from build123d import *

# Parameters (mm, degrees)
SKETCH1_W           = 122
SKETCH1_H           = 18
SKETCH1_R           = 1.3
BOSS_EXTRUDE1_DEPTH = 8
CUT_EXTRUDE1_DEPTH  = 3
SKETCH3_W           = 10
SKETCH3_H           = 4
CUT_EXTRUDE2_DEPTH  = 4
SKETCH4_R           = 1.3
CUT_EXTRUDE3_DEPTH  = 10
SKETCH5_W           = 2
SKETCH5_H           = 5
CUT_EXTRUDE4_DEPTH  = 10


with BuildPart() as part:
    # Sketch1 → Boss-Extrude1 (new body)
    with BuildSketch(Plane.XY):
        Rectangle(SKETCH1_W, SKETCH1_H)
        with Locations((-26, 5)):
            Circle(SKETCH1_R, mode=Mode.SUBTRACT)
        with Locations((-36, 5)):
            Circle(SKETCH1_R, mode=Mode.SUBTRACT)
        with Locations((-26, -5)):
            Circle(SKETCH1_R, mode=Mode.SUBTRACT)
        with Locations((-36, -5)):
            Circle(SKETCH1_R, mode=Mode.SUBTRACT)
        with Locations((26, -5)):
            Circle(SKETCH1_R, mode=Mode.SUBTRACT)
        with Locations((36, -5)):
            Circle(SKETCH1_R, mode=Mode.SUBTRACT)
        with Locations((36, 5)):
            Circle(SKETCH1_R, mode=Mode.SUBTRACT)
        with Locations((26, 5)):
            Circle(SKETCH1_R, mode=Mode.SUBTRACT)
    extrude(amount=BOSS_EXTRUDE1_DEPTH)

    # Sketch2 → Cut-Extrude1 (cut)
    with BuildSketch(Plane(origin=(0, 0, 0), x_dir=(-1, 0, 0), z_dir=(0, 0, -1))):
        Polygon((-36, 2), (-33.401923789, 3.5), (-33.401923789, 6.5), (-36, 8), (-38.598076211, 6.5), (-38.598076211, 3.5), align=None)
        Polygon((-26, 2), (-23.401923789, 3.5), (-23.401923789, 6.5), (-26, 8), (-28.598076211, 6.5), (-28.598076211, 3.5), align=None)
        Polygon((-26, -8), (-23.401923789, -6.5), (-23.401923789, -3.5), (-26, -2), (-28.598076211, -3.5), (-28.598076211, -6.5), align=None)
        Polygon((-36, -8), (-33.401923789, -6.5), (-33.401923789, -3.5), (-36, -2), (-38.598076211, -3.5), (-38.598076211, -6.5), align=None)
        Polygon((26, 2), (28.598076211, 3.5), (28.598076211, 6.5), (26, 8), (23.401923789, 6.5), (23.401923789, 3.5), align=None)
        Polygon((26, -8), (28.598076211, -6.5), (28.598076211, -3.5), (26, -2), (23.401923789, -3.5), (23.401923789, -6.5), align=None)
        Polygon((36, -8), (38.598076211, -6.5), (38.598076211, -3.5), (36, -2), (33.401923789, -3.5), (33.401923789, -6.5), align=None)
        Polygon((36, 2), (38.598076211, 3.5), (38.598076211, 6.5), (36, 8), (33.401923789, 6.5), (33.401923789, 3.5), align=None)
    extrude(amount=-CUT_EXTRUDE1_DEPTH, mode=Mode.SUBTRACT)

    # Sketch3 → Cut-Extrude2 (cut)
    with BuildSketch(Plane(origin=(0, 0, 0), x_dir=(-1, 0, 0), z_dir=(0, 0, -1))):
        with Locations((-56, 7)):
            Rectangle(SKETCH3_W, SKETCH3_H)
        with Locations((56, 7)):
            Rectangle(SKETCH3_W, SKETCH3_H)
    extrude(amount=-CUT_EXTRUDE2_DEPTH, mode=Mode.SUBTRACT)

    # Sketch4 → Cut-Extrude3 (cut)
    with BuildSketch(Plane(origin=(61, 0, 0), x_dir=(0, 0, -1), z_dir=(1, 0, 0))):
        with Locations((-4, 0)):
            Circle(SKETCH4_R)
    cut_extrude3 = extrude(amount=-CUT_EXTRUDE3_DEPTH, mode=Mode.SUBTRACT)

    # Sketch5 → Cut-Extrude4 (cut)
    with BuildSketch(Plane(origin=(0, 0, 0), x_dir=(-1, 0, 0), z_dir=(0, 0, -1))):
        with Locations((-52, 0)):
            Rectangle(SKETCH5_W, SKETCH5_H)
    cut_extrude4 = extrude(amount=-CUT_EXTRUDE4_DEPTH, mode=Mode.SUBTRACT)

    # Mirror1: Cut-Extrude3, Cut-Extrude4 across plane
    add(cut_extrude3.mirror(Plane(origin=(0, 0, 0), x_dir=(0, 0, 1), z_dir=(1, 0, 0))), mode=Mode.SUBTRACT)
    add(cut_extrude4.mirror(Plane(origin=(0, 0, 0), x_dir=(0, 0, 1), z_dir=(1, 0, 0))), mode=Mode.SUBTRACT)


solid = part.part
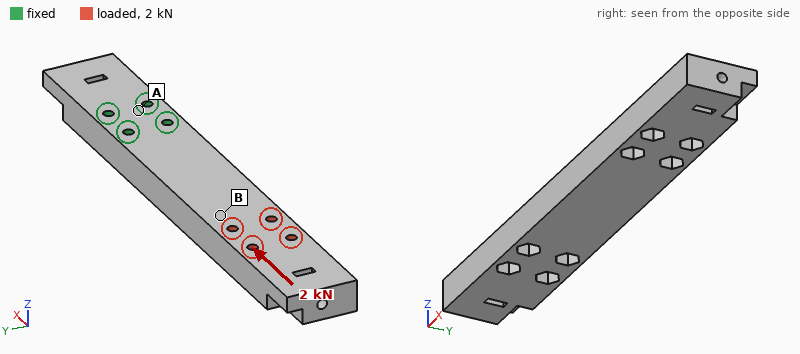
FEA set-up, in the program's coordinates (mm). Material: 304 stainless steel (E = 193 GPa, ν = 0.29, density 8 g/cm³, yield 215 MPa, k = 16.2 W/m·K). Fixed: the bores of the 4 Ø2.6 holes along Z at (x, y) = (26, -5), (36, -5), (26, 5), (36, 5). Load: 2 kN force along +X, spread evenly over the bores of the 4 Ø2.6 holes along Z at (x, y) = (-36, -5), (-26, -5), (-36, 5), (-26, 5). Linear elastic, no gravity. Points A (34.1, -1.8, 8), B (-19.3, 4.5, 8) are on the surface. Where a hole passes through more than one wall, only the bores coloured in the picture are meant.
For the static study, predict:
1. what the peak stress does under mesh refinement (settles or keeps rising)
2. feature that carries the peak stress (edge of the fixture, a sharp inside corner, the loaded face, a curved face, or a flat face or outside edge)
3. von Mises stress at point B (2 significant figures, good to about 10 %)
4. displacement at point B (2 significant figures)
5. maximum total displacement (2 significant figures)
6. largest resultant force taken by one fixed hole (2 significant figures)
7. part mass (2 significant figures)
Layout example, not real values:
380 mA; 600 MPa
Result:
keeps rising; edge of the fixture; 29 MPa; 21 µm; 65 µm; 880 N; 130 g
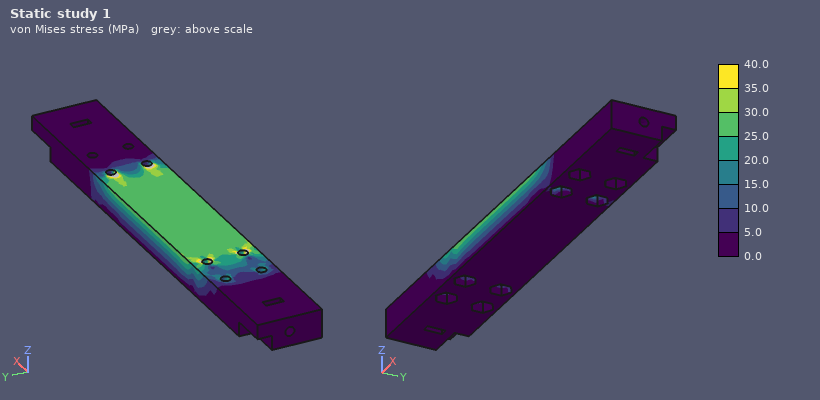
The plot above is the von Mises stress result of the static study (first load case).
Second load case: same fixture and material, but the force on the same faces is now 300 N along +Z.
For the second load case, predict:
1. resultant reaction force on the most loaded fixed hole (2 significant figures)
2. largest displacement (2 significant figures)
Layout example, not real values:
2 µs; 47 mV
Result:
640 N; 0.27 mm
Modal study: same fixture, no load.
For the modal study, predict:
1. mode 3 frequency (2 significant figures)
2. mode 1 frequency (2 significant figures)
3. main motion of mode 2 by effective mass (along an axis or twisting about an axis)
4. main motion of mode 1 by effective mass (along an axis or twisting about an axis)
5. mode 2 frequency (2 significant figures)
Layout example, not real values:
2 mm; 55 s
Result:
4600 Hz; 800 Hz; along Y; along Z; 1800 Hz
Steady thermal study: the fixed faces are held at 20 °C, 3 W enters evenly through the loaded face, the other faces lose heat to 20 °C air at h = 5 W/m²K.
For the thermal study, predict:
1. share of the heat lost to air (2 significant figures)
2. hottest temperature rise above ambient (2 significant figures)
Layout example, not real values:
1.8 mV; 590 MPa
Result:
32 %; 57 K
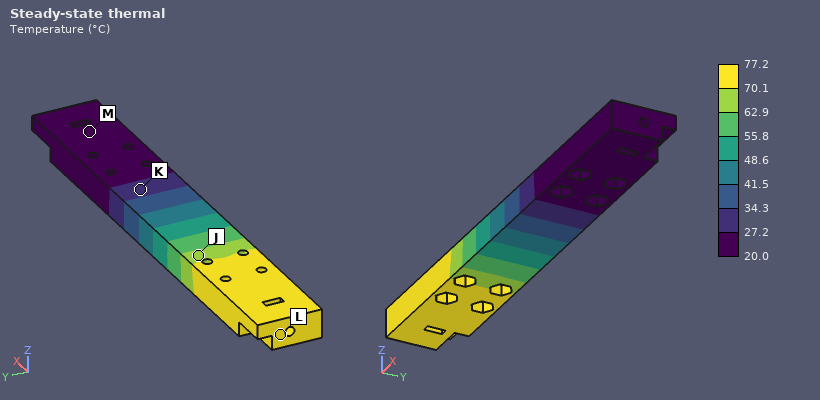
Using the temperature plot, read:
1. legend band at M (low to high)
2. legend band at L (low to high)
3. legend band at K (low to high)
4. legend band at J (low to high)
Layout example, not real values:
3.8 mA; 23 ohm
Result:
20.0 to 27.2 °C; 70.1 to 77.2 °C; 27.2 to 34.3 °C; 62.9 to 70.1 °C
